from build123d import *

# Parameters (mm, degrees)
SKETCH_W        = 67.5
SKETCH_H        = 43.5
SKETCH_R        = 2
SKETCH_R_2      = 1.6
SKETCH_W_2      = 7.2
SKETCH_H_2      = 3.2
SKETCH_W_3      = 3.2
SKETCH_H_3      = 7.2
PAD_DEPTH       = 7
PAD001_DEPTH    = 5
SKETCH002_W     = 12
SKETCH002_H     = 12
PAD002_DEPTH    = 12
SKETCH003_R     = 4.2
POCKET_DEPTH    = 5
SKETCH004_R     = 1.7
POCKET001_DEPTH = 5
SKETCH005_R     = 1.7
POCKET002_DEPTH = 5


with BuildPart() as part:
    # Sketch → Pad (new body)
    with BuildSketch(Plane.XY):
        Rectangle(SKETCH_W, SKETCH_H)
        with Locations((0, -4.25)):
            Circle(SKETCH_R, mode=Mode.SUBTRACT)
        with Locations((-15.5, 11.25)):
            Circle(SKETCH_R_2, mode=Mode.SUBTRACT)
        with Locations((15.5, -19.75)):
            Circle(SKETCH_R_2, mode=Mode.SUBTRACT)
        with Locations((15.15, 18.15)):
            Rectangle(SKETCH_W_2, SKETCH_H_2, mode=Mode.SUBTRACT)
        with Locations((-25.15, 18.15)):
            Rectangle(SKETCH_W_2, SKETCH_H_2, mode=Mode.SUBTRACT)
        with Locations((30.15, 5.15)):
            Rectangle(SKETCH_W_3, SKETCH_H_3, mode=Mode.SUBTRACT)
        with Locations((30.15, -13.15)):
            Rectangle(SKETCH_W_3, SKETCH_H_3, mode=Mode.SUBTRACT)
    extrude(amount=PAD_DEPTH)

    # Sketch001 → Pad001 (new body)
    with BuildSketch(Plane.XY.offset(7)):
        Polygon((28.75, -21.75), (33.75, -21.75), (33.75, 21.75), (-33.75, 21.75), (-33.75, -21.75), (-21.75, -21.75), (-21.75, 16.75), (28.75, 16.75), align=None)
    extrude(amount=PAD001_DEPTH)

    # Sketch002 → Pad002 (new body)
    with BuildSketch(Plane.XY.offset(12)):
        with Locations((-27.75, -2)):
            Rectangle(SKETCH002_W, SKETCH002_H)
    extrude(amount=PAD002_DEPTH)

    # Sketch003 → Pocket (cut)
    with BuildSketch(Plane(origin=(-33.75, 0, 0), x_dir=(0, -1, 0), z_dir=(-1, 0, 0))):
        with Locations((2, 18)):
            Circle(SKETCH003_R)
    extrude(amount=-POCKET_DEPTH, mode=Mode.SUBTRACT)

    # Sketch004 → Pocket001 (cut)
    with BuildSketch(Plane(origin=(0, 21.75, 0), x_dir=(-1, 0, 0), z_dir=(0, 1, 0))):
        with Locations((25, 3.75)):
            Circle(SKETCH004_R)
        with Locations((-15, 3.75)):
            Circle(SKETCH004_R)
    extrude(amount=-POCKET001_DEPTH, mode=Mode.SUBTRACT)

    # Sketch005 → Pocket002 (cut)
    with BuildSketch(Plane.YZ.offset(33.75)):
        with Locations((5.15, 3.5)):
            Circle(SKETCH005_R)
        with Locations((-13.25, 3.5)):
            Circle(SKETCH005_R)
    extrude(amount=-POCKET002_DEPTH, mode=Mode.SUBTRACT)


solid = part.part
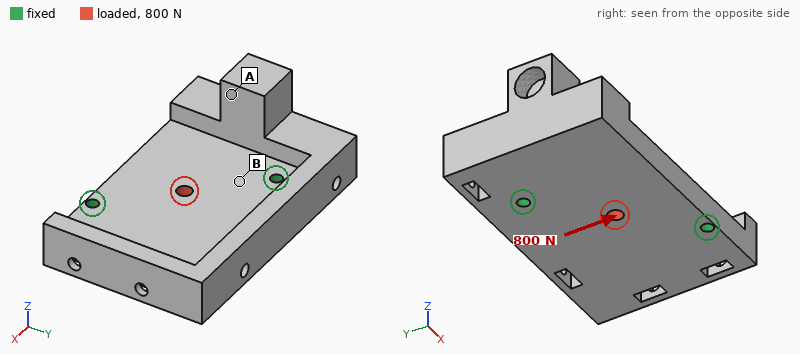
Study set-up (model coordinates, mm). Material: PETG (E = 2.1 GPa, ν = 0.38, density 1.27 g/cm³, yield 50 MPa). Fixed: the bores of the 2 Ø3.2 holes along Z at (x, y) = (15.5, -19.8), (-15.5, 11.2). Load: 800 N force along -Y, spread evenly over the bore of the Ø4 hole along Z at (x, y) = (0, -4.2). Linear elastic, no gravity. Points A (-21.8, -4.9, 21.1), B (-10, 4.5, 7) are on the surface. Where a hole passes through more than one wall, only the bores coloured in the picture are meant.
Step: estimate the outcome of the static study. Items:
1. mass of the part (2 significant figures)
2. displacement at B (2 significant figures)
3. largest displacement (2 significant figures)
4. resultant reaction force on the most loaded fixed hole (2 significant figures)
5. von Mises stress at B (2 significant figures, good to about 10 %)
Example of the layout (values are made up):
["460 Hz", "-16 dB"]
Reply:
["33 g", "26 µm", "73 µm", "410 N", "4.1 MPa"]
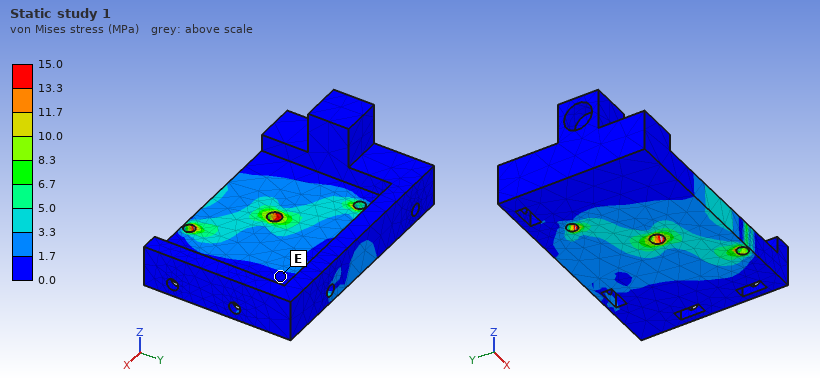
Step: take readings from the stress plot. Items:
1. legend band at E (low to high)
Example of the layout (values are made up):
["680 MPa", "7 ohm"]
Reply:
["0.0 to 1.7 MPa"]
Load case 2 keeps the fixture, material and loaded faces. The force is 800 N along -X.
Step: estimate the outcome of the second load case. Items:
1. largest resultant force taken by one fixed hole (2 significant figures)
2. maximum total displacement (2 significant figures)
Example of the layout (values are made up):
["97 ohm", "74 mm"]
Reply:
["420 N", "66 µm"]
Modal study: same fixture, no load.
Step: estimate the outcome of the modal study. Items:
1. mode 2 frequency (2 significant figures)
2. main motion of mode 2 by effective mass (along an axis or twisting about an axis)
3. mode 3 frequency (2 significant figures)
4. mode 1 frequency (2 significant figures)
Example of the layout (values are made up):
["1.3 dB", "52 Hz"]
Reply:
["1300 Hz", "along Z", "2200 Hz", "860 Hz"]
